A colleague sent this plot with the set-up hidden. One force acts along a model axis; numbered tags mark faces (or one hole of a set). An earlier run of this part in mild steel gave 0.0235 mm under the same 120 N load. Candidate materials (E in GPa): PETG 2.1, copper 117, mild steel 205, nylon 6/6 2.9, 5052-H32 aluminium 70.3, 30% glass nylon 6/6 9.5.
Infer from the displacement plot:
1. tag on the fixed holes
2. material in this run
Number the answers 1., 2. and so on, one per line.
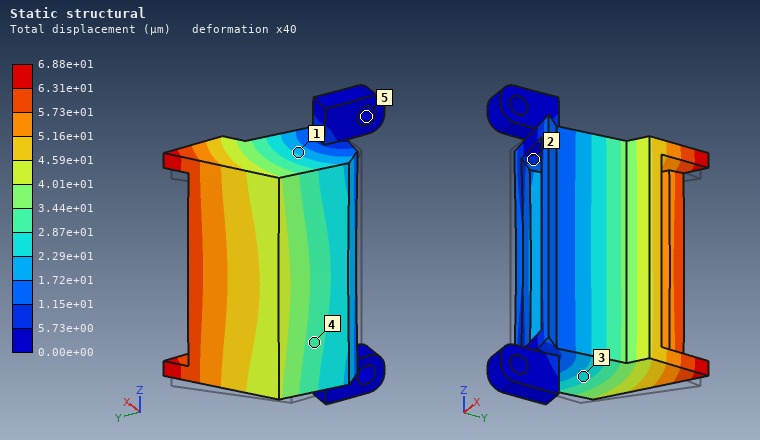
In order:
1. 5
2. 5052-H32 aluminium
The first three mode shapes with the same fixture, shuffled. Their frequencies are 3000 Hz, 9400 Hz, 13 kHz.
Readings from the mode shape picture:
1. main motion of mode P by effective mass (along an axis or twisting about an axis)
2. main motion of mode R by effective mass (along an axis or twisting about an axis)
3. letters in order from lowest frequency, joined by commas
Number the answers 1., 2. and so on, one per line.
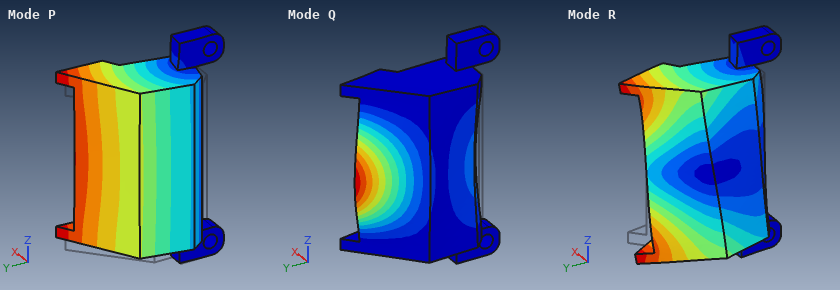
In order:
1. along X
2. twisting about Y
3. P, R, Q
